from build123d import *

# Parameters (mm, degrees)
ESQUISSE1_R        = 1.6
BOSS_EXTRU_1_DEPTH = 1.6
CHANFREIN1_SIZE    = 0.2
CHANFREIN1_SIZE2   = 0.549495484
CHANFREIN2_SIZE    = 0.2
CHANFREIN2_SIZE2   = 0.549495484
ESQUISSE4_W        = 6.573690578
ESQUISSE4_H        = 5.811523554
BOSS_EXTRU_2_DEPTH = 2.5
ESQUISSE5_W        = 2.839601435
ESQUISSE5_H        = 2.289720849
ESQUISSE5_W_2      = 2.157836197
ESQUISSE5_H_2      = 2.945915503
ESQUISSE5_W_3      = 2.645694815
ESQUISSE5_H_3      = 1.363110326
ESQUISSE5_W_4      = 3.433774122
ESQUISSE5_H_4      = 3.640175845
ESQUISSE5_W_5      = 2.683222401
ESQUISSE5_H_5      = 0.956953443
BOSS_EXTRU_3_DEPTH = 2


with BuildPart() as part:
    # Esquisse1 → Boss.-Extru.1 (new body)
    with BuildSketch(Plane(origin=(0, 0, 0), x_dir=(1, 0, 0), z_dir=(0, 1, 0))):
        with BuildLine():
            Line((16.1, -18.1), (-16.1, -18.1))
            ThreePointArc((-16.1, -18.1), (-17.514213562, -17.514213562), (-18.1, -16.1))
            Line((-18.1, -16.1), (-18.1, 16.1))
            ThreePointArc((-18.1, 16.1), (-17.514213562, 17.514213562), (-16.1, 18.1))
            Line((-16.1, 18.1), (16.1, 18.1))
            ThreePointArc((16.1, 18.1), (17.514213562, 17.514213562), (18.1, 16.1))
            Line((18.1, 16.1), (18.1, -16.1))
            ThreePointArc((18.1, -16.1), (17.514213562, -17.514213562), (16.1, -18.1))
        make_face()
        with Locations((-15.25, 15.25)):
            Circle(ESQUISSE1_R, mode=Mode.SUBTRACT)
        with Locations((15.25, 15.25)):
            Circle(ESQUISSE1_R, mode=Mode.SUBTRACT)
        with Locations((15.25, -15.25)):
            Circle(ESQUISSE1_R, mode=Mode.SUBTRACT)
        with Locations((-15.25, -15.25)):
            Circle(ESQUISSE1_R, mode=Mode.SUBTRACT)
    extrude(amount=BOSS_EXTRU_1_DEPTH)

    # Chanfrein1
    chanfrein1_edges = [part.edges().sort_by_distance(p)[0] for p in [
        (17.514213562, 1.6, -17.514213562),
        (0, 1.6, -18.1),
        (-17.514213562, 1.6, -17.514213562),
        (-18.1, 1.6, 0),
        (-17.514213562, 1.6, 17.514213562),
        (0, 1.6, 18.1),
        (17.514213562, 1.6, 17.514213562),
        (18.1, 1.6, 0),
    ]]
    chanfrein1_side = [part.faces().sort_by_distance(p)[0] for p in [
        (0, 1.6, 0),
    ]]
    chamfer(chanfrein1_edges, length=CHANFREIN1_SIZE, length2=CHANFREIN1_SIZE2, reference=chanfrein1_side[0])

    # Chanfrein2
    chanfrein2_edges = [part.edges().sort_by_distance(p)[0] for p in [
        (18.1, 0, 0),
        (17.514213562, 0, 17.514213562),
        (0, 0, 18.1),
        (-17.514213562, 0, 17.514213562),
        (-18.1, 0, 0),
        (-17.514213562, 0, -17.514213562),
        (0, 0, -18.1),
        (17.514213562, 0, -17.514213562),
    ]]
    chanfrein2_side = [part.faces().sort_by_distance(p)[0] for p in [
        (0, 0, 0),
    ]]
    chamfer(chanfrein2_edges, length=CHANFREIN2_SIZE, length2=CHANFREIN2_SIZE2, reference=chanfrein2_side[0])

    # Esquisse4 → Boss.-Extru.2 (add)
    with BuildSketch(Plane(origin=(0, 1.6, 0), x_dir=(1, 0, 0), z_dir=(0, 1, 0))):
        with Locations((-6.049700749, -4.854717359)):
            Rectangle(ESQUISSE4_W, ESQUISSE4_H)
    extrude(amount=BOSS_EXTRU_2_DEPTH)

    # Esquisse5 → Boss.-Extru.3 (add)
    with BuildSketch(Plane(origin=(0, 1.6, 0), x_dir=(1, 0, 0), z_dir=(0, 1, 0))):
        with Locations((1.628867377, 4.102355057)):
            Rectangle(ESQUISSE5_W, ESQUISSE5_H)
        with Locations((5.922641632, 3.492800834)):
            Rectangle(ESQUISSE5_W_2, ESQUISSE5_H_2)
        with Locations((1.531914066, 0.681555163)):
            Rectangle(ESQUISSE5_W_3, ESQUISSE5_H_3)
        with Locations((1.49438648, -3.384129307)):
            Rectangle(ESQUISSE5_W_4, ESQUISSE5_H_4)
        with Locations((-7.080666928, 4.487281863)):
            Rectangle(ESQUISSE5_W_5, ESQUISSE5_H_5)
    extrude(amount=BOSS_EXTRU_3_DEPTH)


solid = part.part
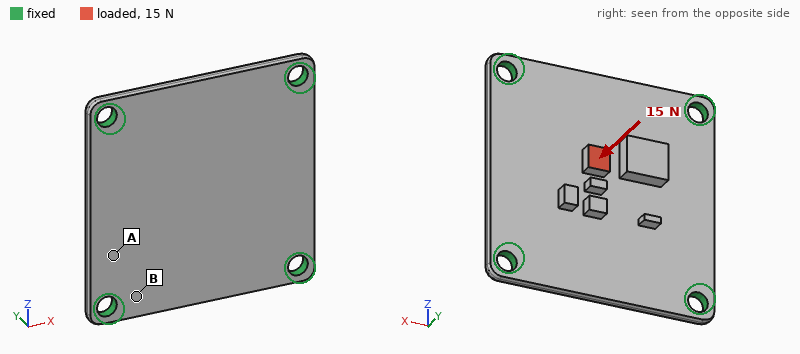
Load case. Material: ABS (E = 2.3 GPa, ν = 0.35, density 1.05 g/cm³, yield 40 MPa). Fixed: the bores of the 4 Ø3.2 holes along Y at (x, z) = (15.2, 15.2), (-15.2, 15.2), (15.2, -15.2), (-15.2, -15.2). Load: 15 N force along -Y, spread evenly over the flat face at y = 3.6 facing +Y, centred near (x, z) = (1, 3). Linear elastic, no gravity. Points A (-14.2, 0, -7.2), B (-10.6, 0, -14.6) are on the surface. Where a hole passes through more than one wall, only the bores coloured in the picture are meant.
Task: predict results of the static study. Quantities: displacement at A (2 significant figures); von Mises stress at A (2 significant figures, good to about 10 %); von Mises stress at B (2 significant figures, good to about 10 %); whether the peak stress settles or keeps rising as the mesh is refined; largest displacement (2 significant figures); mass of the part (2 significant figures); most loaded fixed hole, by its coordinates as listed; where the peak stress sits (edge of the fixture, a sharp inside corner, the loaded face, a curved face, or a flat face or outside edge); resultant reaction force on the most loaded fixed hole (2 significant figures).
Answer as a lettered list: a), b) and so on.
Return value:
a) 0.029 mm
b) 1.4 MPa
c) 2.3 MPa
d) keeps rising
e) 0.17 mm
f) 2.3 g
g) (15.2, 15.2)
h) edge of the fixture
i) 5.4 N
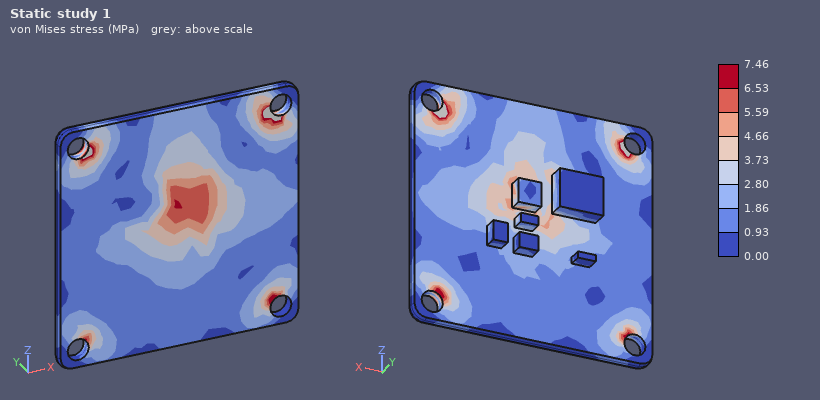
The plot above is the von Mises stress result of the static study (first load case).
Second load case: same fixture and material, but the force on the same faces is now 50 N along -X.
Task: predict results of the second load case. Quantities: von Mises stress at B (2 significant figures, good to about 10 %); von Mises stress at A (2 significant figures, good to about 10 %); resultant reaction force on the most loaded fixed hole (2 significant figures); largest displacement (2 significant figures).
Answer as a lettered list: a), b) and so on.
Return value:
a) 1.3 MPa
b) 0.70 MPa
c) 17 N
d) 100 µm
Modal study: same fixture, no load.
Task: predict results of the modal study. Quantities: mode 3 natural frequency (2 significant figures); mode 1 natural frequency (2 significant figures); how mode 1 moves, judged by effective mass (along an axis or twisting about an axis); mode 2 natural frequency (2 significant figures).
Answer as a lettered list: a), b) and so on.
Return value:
a) 3300 Hz
b) 1800 Hz
c) along Y
d) 3200 Hz
